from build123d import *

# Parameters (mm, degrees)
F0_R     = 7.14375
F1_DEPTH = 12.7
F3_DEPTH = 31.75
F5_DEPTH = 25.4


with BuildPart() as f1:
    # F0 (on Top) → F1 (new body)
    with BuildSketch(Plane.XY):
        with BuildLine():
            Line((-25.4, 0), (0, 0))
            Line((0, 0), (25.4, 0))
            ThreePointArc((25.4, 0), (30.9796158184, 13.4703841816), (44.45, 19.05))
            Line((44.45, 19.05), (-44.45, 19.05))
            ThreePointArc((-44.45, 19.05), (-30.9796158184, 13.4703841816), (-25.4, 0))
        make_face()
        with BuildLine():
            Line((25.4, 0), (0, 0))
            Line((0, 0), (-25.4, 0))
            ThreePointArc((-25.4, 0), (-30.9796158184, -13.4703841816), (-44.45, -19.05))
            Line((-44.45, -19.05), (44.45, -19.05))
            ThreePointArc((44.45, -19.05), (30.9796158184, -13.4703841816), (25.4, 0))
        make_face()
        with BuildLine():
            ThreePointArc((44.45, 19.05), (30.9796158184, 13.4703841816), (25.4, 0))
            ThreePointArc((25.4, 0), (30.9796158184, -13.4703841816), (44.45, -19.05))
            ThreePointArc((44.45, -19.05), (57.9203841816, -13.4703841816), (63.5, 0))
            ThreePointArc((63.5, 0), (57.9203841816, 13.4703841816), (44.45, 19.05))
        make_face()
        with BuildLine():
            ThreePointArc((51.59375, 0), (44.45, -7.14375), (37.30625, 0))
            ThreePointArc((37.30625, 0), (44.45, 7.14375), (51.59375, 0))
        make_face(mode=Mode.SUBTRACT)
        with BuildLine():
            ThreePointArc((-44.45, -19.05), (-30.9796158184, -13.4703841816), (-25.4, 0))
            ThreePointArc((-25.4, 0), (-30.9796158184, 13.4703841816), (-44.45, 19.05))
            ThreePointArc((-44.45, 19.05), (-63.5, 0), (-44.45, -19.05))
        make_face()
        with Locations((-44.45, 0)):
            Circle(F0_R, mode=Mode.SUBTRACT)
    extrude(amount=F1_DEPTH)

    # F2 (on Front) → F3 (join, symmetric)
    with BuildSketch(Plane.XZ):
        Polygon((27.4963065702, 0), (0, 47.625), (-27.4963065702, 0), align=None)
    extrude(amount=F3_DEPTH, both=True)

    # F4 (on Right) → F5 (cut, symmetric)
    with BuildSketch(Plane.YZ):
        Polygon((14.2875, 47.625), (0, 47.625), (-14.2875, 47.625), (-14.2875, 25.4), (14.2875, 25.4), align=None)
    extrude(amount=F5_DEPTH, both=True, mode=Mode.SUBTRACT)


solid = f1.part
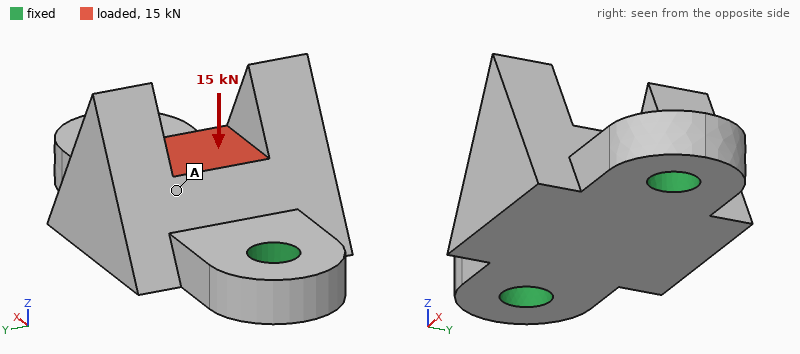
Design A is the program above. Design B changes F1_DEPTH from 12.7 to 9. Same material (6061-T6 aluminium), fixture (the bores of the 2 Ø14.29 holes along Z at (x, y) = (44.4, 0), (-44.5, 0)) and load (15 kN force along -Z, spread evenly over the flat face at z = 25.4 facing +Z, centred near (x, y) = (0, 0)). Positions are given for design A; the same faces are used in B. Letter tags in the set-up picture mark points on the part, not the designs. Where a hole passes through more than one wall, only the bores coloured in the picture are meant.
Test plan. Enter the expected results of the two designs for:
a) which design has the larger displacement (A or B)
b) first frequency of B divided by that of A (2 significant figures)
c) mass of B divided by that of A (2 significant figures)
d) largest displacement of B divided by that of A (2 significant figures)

B
0.69
0.91
1.6
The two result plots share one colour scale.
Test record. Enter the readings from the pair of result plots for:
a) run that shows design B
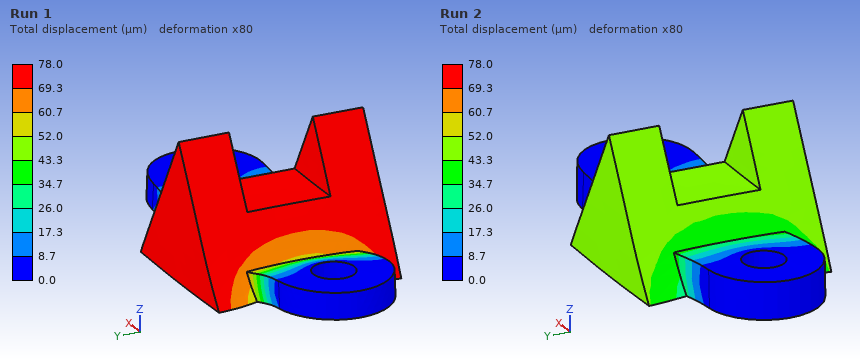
Run 1
